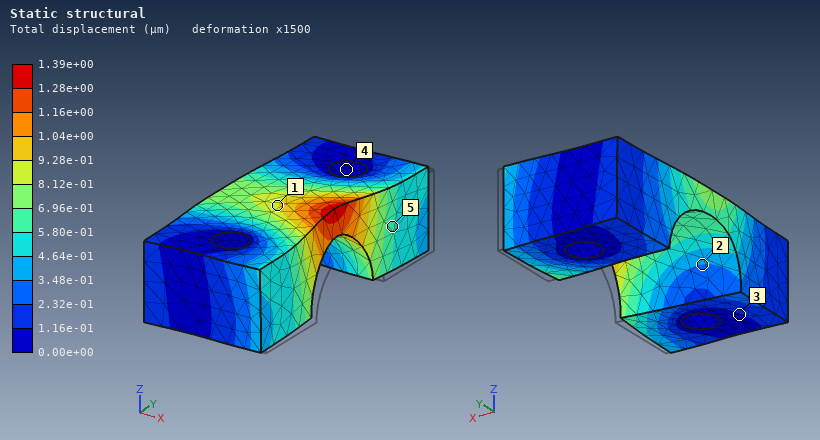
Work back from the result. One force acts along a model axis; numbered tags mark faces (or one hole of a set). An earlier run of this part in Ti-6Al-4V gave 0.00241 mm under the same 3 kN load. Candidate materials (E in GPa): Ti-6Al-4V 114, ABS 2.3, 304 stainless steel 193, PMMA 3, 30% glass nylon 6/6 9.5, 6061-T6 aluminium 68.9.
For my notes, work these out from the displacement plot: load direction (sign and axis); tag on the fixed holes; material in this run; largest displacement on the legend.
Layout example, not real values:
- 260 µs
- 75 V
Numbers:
- -X
- 4
- 304 stainless steel
- 1.39e+00 µm
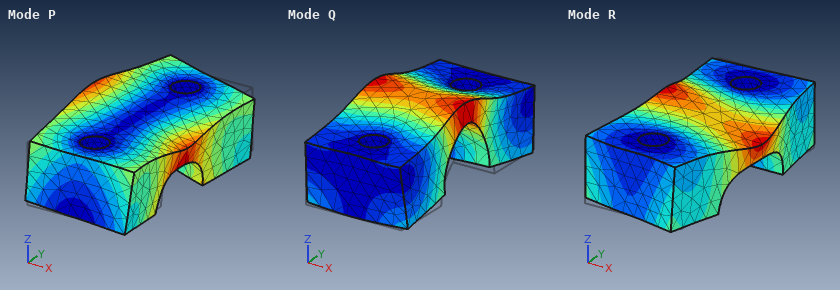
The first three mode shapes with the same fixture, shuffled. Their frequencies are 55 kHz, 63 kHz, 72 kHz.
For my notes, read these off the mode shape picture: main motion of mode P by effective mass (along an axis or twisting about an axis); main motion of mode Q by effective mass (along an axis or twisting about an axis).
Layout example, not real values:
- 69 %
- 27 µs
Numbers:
- twisting about Y
- along Z
